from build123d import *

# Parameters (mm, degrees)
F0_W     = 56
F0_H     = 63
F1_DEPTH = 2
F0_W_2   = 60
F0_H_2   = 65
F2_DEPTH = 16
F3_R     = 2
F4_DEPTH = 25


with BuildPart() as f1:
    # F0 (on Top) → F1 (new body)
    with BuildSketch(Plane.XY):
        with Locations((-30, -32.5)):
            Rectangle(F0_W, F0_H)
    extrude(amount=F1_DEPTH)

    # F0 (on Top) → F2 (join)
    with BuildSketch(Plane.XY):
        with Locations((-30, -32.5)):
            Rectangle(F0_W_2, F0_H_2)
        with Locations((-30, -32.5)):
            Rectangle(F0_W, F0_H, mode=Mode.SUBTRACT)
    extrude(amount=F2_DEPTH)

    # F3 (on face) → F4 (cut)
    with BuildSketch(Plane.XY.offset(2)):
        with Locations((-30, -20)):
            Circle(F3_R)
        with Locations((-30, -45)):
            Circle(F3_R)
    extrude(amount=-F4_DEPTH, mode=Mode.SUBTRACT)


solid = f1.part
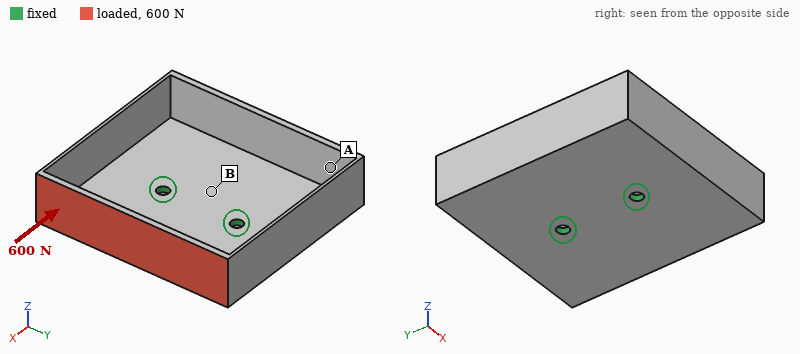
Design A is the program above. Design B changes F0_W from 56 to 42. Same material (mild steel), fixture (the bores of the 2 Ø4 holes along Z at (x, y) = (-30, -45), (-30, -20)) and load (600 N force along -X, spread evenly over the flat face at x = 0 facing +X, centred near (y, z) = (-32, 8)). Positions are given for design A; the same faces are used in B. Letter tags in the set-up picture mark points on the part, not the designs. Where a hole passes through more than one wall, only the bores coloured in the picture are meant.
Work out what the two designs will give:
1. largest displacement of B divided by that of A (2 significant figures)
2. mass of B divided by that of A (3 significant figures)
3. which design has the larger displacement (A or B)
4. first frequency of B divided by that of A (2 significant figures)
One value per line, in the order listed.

0.52
1.95
A
0.72
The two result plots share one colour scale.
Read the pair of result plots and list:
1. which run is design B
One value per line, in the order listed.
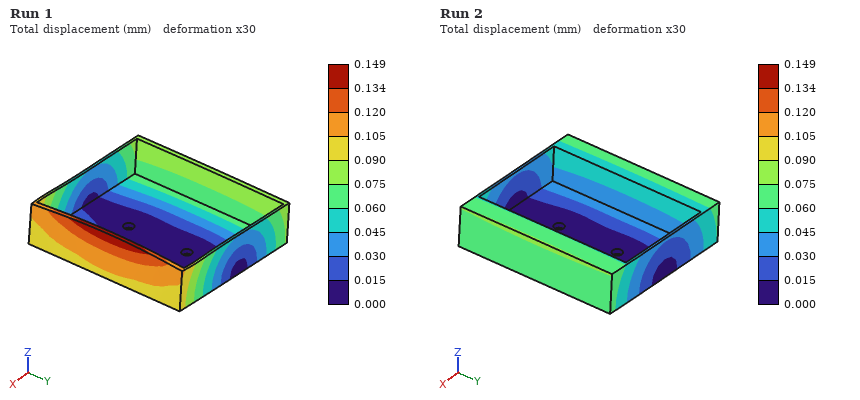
Run 2
